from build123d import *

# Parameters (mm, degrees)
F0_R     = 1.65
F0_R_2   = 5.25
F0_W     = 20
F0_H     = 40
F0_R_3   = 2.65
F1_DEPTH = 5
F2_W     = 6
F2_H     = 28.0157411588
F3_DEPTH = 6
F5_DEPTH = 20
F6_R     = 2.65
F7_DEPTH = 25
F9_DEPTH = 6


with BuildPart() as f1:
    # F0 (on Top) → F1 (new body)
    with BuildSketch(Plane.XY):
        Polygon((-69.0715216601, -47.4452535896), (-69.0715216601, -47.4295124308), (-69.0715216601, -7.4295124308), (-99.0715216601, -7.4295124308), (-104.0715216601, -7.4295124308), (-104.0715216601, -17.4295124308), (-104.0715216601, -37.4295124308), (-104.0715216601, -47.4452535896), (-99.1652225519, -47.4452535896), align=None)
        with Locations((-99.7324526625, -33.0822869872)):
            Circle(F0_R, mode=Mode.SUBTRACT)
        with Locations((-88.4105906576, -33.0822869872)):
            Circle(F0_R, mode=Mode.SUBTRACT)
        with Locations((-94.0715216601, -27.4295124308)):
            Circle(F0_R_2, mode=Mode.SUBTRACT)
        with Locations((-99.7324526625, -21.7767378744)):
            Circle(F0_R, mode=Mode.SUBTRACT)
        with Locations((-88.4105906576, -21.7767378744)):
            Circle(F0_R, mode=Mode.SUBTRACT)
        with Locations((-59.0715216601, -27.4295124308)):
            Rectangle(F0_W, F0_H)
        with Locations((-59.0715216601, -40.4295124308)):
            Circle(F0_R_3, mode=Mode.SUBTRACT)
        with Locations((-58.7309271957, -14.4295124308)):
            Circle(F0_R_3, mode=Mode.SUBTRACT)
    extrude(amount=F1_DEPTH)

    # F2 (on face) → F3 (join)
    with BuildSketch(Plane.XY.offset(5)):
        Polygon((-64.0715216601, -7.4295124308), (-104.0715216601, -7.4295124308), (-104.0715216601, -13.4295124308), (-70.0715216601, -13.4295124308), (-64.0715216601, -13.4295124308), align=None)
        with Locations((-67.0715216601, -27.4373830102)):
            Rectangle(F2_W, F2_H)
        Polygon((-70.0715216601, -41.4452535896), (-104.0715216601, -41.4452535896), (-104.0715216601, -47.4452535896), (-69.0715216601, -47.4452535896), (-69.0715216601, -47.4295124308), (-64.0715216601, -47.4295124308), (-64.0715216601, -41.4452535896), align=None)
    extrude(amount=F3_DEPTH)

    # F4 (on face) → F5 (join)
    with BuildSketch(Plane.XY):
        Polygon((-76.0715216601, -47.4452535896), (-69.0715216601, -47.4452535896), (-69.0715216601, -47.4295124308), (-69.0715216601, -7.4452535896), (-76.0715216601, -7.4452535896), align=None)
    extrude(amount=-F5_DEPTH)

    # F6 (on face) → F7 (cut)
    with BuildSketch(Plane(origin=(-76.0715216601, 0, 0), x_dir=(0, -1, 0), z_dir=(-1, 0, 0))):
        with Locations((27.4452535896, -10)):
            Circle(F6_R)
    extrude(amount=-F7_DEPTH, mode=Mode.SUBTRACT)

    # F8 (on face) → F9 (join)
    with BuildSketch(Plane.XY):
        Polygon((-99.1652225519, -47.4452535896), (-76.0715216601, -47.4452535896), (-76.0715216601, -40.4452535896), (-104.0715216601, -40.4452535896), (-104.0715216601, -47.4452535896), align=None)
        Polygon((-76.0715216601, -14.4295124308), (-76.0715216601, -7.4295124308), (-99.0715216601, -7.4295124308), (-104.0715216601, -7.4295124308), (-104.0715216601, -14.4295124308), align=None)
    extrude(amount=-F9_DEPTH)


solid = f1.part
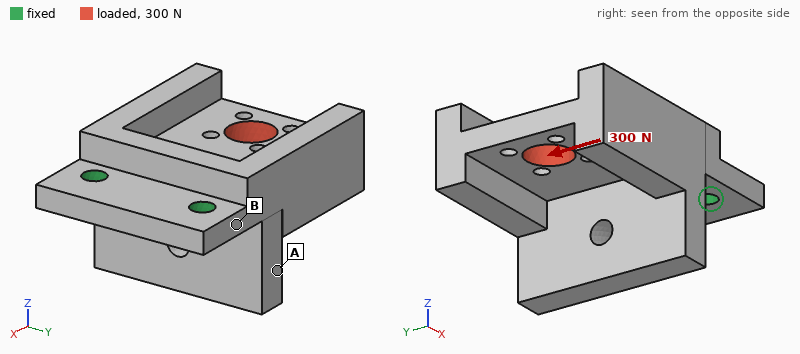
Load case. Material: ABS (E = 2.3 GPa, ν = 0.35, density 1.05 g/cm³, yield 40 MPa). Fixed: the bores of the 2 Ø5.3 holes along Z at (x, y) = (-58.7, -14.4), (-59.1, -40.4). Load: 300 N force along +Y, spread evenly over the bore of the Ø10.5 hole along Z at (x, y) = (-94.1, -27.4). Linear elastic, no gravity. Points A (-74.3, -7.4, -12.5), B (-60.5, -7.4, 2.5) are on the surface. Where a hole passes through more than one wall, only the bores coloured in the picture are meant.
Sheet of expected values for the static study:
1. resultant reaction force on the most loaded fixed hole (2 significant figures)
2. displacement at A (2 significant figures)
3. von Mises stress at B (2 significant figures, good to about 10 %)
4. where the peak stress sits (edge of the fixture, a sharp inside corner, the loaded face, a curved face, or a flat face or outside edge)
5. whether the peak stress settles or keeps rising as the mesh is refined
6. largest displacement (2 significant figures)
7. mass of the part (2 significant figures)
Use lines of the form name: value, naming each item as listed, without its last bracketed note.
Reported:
resultant reaction force on the most loaded fixed hole: 400 N
displacement at A: 0.069 mm
von Mises stress at B: 4.9 MPa
where the peak stress sits: edge of the fixture
whether the peak stress settles or keeps rising as the mesh is refined: keeps rising
largest displacement: 0.19 mm
mass of the part: 23 g
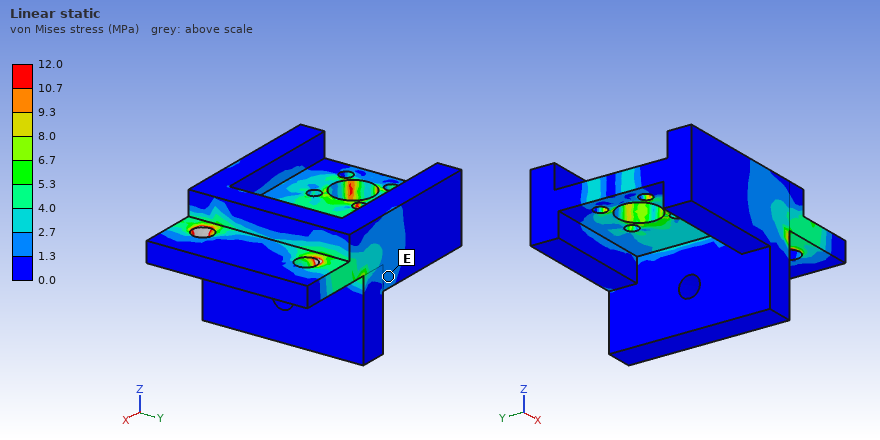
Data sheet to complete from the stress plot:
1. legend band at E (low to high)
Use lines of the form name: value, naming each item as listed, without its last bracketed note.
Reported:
legend band at E: 1.3 to 2.7 MPa
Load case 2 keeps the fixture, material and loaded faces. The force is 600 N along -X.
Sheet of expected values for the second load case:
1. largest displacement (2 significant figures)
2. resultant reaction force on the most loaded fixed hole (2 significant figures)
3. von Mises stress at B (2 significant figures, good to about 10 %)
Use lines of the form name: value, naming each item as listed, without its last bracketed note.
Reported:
largest displacement: 0.11 mm
resultant reaction force on the most loaded fixed hole: 300 N
von Mises stress at B: 2.1 MPa
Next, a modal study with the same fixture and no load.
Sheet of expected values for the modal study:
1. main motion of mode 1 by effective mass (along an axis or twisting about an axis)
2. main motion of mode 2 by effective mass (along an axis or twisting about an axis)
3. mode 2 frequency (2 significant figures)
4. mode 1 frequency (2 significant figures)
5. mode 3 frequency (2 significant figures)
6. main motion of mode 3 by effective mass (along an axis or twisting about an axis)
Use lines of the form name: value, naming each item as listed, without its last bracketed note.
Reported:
main motion of mode 1 by effective mass: along Z
main motion of mode 2 by effective mass: twisting about X
mode 2 frequency: 1400 Hz
mode 1 frequency: 560 Hz
mode 3 frequency: 2400 Hz
main motion of mode 3 by effective mass: along Y
